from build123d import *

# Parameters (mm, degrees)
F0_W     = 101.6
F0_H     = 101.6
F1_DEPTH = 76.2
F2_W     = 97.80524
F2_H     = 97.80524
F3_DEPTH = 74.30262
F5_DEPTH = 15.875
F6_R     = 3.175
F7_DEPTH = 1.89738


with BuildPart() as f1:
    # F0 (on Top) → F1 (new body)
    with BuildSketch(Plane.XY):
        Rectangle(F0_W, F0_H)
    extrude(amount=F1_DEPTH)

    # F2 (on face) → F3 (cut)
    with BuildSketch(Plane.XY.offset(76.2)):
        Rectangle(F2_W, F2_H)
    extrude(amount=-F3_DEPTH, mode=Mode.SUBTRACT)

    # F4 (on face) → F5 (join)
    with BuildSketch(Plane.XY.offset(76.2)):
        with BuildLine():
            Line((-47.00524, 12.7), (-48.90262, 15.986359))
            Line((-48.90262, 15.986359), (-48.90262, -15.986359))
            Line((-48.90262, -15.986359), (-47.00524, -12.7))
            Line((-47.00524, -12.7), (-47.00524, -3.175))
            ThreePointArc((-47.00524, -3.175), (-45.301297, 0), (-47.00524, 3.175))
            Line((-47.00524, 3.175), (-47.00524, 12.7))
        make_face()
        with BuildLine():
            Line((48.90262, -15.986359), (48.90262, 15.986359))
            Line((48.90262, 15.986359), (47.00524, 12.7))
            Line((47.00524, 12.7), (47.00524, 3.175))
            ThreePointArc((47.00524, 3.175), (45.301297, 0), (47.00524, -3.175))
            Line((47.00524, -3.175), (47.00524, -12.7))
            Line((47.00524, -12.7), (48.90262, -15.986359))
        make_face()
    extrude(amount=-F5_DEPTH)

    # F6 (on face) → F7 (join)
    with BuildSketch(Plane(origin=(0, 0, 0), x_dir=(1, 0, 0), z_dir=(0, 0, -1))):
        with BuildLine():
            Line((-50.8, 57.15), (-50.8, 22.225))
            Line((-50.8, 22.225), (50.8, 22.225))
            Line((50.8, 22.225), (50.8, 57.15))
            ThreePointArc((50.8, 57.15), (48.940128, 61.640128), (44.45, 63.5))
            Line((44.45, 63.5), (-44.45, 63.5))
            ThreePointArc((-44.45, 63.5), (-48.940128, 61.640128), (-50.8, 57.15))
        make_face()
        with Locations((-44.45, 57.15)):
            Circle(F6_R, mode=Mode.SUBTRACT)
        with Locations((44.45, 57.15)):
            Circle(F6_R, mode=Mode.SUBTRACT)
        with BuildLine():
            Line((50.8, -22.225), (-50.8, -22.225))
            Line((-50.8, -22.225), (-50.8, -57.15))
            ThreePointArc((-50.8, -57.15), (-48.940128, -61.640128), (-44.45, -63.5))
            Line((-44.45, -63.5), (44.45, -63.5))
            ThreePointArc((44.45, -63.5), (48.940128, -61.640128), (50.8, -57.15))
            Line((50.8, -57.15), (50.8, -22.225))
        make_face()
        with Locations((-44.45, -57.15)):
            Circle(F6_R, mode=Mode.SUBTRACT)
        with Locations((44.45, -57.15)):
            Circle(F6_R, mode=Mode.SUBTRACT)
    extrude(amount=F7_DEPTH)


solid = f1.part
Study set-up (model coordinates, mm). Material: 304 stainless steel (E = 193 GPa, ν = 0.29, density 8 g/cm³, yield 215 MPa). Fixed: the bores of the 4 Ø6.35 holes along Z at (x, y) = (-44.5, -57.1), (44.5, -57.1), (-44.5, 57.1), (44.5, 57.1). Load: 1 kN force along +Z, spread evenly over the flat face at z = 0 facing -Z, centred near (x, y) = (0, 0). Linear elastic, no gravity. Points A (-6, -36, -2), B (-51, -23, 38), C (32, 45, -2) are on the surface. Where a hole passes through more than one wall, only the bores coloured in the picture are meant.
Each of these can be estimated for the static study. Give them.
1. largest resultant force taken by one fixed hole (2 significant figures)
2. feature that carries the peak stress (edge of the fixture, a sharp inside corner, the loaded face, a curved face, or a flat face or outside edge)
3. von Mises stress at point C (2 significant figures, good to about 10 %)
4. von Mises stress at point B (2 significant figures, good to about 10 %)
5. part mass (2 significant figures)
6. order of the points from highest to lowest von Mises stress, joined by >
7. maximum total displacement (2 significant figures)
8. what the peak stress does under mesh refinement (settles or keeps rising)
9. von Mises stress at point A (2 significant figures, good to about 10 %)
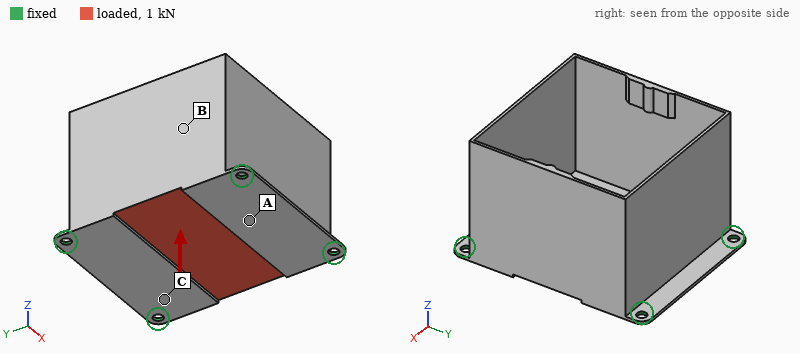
720 N
edge of the fixture
35 MPa
6.9 MPa
750 g
C > A > B
0.12 mm
keeps rising
18 MPa
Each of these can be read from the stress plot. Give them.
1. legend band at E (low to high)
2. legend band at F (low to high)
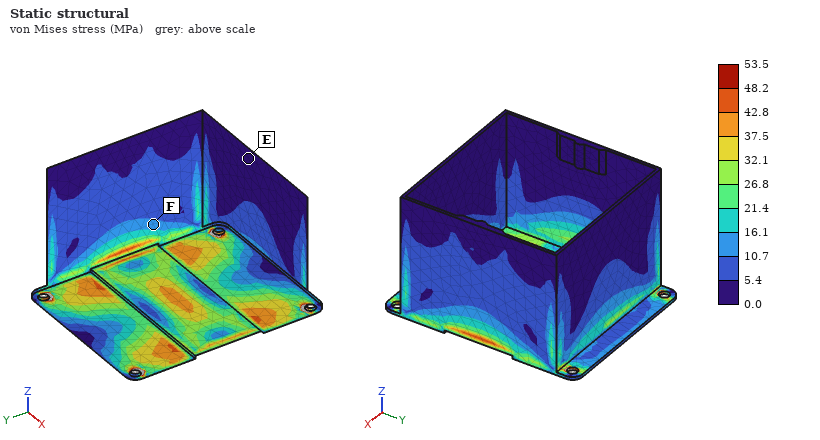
0.0 to 5.4 MPa
10.7 to 16.1 MPa
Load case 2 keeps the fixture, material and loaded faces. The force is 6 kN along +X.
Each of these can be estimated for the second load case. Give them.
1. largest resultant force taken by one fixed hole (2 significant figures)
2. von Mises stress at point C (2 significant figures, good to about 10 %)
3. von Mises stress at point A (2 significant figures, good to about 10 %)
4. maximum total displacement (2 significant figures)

1.7 kN
19 MPa
16 MPa
11 µm
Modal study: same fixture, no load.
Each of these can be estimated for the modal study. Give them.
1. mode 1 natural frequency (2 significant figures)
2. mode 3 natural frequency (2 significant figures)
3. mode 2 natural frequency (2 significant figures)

670 Hz
880 Hz
860 Hz
